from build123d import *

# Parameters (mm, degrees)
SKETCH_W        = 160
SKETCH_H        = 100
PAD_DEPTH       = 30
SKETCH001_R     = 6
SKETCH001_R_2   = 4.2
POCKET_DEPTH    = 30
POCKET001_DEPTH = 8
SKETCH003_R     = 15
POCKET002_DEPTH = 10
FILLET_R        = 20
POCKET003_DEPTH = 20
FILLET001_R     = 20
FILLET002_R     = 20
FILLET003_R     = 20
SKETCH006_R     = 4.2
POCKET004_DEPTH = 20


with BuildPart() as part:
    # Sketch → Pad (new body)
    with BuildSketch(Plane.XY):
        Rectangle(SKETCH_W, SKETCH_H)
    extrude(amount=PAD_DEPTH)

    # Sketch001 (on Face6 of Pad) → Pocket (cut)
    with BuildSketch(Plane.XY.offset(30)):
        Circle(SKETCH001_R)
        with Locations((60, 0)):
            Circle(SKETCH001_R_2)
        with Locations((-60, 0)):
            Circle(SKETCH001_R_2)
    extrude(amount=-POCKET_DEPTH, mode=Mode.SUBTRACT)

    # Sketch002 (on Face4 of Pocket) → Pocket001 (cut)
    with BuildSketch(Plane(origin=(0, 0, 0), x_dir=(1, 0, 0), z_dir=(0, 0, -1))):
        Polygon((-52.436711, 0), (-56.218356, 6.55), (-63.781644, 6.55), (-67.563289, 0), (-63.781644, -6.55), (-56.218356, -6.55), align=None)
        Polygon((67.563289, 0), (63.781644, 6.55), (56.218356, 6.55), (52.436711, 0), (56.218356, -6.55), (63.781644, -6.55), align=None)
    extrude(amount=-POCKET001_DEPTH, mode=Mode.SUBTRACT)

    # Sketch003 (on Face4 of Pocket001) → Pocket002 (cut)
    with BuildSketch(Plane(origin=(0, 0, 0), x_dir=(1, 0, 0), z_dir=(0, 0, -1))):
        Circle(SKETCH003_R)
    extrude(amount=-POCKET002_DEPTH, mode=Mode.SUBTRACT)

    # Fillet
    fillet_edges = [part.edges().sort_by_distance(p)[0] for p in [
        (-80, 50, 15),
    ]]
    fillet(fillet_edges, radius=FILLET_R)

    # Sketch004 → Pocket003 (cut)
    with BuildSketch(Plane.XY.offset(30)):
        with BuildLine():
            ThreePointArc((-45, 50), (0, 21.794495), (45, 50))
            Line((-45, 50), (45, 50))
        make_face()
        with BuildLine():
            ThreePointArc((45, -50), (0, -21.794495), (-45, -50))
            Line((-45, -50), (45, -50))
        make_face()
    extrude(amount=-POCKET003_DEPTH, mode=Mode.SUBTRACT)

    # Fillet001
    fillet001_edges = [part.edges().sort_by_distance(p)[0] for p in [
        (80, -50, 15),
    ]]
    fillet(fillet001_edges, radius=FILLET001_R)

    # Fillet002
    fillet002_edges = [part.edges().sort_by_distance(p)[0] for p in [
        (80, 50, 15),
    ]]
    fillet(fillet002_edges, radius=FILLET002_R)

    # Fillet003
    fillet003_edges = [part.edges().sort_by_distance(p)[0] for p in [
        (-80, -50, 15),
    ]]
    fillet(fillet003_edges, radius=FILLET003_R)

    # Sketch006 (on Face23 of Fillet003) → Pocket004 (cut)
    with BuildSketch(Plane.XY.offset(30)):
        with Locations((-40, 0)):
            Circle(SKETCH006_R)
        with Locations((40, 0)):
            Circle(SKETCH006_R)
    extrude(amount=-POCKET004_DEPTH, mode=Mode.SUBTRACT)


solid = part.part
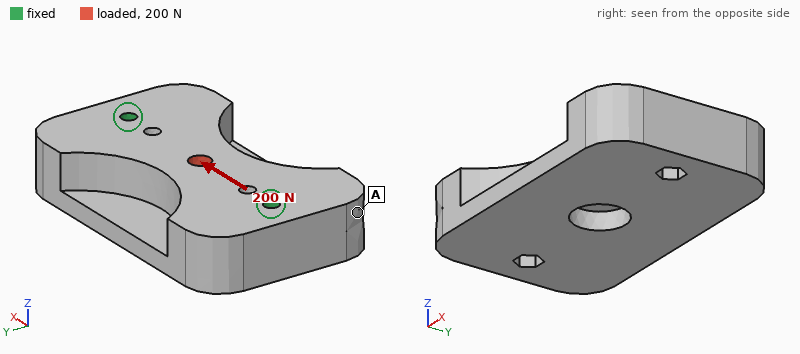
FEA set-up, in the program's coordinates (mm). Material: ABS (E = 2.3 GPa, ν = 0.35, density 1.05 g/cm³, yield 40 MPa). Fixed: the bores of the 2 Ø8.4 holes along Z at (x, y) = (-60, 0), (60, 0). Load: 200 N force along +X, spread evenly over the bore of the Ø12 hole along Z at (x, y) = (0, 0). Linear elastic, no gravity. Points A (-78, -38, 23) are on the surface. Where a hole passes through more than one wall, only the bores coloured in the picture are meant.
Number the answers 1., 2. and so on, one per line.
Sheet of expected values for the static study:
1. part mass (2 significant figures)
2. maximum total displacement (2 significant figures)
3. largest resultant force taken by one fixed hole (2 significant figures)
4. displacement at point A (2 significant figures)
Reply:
1. 400 g
2. 3.9 µm
3. 100 N
4. 1.4 µm
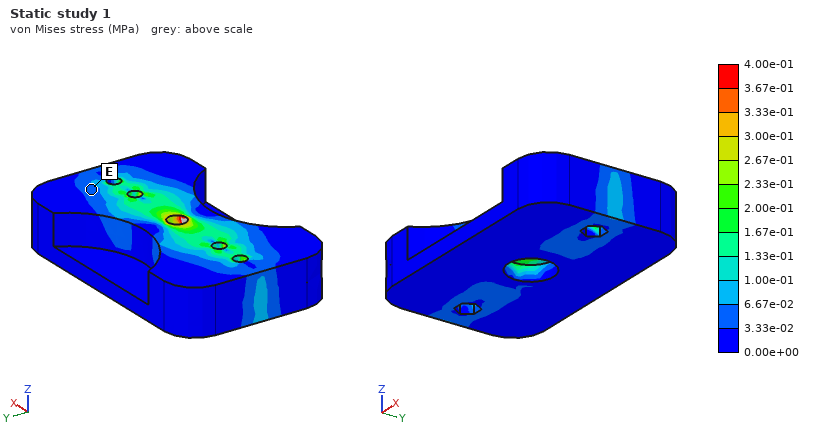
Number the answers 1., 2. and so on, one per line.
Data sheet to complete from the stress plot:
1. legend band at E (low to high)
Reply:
1. 3.33e-02 to 6.67e-02 MPa
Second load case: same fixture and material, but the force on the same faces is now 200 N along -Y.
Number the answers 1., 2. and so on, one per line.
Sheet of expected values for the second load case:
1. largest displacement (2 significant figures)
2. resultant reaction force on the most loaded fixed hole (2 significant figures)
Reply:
1. 9.7 µm
2. 100 N
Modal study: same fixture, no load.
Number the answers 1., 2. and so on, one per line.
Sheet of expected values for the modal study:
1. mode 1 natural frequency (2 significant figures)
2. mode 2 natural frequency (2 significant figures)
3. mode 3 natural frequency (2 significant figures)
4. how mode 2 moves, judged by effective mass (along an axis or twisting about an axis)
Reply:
1. 1100 Hz
2. 1500 Hz
3. 1700 Hz
4. along Z
